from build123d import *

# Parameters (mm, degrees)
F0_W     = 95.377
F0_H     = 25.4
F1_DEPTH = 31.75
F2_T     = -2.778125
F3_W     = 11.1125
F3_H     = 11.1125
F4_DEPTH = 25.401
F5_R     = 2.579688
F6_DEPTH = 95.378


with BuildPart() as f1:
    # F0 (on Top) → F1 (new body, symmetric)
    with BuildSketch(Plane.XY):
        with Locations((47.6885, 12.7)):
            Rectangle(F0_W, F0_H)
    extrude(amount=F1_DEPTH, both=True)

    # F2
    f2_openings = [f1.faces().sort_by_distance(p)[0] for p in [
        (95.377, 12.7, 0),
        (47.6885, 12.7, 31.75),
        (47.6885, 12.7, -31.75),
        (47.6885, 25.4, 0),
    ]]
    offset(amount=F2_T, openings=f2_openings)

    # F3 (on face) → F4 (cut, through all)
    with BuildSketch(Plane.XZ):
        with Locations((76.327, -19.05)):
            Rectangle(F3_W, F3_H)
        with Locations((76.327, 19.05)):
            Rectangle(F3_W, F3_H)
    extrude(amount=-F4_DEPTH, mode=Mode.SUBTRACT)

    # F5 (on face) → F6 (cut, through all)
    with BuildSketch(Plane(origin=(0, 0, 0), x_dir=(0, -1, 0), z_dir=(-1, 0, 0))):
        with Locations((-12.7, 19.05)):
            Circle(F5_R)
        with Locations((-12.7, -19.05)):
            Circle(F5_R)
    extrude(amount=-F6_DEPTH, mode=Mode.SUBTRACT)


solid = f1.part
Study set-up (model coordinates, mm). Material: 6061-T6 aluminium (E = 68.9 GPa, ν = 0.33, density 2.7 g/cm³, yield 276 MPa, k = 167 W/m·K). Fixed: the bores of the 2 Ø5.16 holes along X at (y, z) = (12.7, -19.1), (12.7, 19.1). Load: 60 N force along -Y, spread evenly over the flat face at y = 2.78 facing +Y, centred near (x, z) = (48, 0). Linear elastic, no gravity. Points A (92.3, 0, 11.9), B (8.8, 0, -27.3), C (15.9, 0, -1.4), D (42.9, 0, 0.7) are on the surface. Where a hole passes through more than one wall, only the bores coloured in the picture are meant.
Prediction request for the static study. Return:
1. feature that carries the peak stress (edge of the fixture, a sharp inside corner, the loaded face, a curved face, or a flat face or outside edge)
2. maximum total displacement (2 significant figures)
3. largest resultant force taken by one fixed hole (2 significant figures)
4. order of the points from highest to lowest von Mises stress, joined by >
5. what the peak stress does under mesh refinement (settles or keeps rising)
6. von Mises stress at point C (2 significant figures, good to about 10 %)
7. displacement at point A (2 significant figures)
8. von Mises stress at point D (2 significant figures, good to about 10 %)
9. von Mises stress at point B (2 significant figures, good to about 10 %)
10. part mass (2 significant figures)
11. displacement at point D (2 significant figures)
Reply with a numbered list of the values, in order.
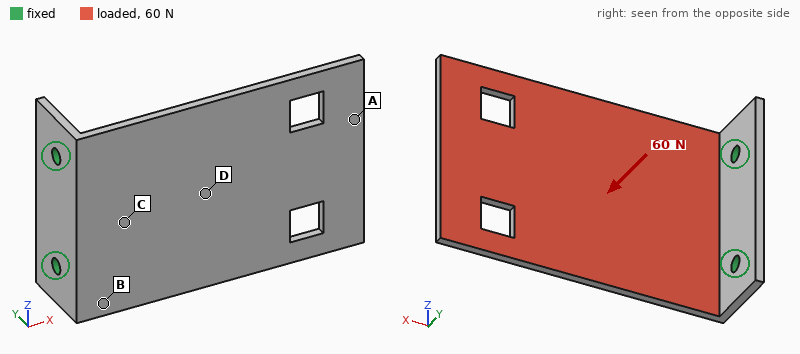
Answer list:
1. edge of the fixture
2. 1.1 mm
3. 31 N
4. B > C > D > A
5. keeps rising
6. 21 MPa
7. 1.0 mm
8. 9.4 MPa
9. 27 MPa
10. 54 g
11. 0.36 mm
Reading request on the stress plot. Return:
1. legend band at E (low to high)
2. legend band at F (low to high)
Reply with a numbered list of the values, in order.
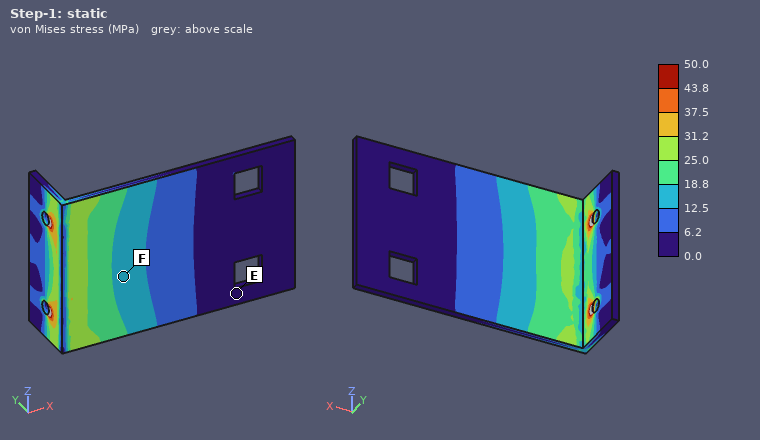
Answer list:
1. 0.0 to 6.2 MPa
2. 12.5 to 18.8 MPa
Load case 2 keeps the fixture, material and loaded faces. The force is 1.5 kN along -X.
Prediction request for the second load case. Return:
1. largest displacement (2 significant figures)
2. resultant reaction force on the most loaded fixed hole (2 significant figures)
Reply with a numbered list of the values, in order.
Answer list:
1. 0.23 mm
2. 750 N
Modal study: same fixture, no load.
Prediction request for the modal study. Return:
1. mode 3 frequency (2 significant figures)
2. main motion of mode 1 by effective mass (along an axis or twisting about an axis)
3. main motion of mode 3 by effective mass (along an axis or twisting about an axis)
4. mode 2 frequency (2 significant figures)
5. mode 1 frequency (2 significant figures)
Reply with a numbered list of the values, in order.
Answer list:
1. 1300 Hz
2. along Y
3. along Z
4. 810 Hz
5. 230 Hz
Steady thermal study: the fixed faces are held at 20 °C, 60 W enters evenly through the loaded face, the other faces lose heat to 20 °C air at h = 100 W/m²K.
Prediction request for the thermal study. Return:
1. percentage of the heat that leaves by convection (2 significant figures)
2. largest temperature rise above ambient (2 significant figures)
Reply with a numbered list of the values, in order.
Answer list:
1. 51 %
2. 56 K
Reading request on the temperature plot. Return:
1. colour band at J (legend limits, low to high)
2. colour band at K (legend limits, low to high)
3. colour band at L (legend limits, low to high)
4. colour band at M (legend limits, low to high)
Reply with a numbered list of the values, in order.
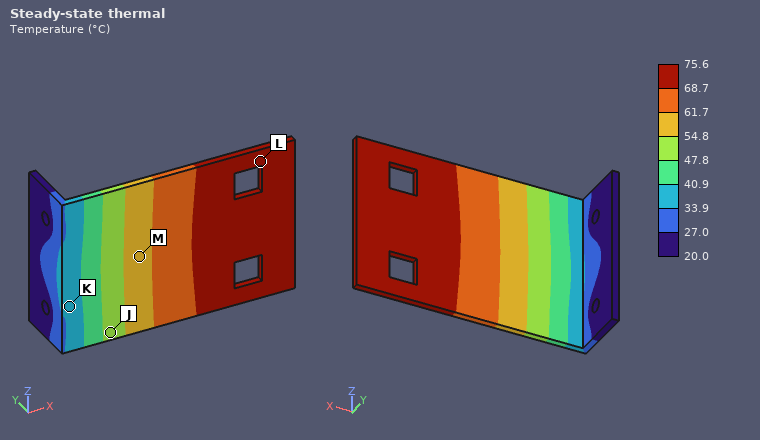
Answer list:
1. 47.8 to 54.8 °C
2. 33.9 to 40.9 °C
3. 68.7 to 75.6 °C
4. 54.8 to 61.7 °C
